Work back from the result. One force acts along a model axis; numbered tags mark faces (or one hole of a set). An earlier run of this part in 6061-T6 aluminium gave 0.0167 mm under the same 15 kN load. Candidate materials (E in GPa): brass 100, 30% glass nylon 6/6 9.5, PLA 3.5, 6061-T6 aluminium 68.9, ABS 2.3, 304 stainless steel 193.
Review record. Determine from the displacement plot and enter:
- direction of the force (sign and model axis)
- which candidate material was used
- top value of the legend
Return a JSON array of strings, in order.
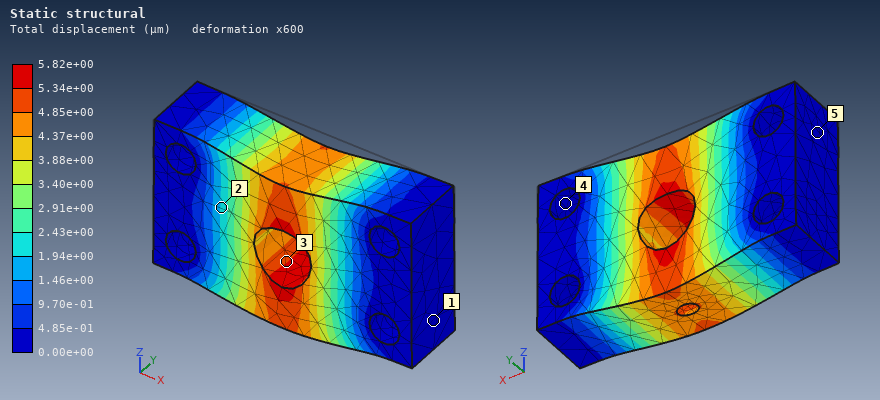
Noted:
["-Z", "304 stainless steel", "5.82e+00 µm"]
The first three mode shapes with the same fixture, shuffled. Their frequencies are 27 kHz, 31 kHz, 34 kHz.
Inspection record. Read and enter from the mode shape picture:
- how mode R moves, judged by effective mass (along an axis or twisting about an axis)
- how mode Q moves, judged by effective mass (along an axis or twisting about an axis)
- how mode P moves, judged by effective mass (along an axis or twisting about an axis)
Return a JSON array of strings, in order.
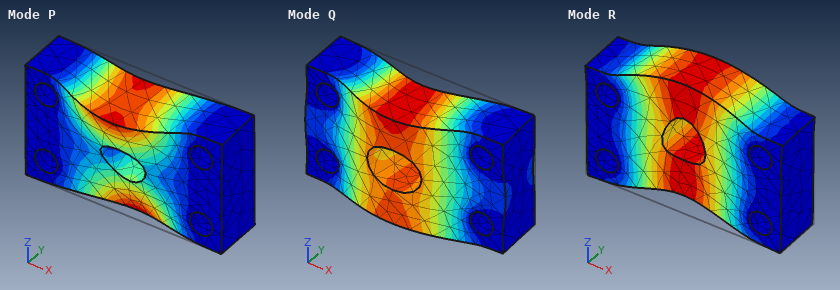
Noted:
["along Z", "along Y", "twisting about X"]
